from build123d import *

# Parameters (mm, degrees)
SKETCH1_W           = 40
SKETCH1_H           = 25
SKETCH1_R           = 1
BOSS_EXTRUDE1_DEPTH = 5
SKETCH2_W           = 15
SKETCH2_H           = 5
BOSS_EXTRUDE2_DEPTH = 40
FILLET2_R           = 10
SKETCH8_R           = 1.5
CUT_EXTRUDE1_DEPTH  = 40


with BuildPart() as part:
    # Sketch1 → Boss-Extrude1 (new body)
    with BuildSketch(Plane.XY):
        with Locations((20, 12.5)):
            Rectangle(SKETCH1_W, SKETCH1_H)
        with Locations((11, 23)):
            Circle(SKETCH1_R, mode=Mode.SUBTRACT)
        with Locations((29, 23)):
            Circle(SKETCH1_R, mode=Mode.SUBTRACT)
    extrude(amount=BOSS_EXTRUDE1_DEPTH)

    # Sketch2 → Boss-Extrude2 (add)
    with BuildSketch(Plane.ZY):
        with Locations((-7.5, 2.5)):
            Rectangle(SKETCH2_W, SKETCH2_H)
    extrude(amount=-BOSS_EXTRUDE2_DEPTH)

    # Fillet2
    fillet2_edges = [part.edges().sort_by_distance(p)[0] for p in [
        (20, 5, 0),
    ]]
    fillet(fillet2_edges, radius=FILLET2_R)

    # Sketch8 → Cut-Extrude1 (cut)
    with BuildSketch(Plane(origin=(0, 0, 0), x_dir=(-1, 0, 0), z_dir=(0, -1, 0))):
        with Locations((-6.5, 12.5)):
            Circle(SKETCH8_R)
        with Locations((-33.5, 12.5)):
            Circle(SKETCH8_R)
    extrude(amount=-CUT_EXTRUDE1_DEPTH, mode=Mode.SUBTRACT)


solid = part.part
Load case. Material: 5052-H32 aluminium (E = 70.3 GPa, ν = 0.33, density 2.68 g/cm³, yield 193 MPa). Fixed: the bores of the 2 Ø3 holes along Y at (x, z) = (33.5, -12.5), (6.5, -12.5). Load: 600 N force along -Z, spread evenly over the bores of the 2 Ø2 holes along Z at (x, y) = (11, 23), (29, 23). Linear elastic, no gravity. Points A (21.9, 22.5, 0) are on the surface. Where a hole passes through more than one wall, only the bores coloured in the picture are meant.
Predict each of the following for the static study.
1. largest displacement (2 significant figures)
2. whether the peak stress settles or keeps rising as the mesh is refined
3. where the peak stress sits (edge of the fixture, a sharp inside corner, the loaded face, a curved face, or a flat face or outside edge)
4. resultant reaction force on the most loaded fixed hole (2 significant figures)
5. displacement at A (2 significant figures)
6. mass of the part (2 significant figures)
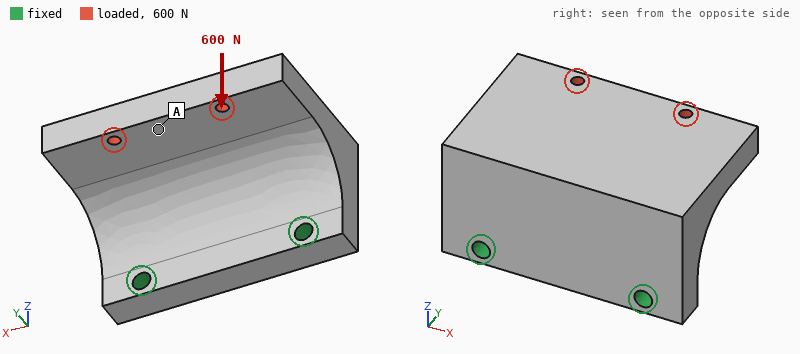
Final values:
0.15 mm
keeps rising
edge of the fixture
330 N
0.12 mm
23 g
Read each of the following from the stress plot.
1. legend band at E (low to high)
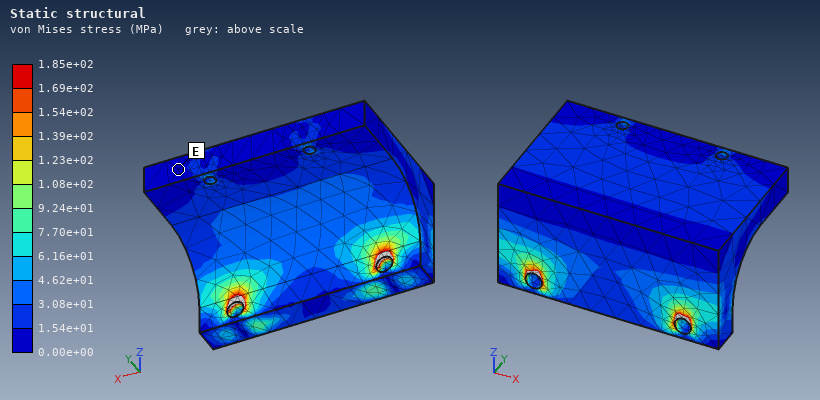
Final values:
0.00e+00 to 1.54e+01 MPa
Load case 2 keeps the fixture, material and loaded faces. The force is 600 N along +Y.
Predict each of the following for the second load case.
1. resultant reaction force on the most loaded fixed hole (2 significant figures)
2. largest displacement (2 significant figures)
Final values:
300 N
74 µm
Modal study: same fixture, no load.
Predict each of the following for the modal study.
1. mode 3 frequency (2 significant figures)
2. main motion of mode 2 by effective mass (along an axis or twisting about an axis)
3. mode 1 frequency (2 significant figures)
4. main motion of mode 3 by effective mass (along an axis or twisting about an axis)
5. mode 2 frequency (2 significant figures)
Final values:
15 kHz
along X
3900 Hz
along Y
8700 Hz
